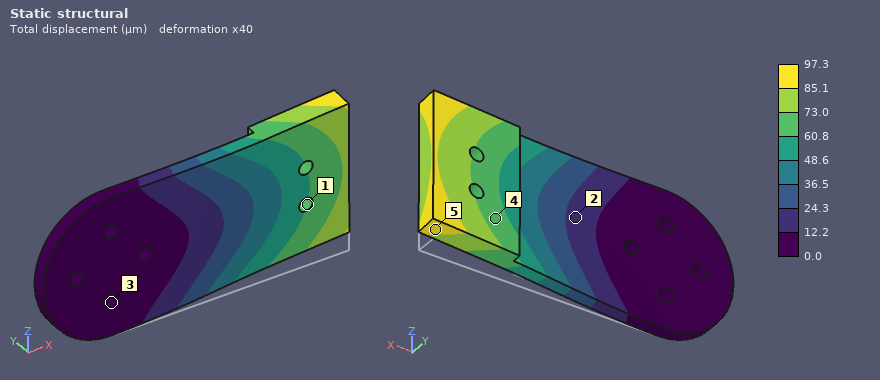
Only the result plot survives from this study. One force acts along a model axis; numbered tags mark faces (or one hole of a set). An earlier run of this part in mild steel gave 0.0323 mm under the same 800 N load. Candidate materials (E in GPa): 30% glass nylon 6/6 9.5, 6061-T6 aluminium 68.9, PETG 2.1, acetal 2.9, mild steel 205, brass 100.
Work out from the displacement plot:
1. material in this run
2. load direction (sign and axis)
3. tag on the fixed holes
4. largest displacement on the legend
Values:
6061-T6 aluminium
+Z
3
97.3 µm
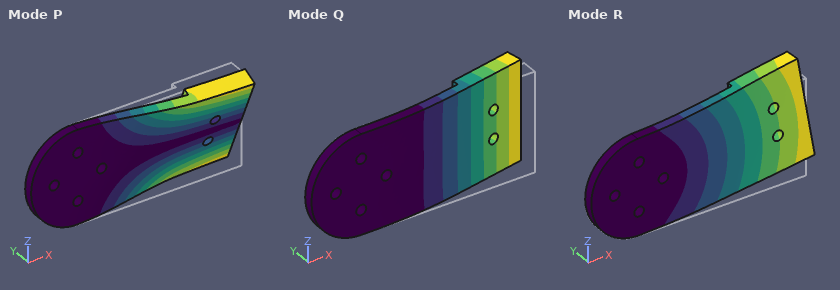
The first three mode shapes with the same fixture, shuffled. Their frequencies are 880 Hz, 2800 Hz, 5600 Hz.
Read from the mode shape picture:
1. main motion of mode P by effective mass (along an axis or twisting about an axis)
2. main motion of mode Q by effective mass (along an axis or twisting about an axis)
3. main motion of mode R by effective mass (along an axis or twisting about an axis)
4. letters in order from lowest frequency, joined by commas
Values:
twisting about X
along Y
along Z
Q, P, R
